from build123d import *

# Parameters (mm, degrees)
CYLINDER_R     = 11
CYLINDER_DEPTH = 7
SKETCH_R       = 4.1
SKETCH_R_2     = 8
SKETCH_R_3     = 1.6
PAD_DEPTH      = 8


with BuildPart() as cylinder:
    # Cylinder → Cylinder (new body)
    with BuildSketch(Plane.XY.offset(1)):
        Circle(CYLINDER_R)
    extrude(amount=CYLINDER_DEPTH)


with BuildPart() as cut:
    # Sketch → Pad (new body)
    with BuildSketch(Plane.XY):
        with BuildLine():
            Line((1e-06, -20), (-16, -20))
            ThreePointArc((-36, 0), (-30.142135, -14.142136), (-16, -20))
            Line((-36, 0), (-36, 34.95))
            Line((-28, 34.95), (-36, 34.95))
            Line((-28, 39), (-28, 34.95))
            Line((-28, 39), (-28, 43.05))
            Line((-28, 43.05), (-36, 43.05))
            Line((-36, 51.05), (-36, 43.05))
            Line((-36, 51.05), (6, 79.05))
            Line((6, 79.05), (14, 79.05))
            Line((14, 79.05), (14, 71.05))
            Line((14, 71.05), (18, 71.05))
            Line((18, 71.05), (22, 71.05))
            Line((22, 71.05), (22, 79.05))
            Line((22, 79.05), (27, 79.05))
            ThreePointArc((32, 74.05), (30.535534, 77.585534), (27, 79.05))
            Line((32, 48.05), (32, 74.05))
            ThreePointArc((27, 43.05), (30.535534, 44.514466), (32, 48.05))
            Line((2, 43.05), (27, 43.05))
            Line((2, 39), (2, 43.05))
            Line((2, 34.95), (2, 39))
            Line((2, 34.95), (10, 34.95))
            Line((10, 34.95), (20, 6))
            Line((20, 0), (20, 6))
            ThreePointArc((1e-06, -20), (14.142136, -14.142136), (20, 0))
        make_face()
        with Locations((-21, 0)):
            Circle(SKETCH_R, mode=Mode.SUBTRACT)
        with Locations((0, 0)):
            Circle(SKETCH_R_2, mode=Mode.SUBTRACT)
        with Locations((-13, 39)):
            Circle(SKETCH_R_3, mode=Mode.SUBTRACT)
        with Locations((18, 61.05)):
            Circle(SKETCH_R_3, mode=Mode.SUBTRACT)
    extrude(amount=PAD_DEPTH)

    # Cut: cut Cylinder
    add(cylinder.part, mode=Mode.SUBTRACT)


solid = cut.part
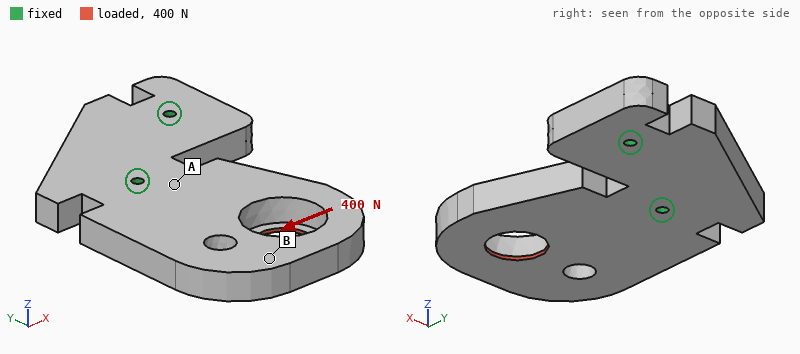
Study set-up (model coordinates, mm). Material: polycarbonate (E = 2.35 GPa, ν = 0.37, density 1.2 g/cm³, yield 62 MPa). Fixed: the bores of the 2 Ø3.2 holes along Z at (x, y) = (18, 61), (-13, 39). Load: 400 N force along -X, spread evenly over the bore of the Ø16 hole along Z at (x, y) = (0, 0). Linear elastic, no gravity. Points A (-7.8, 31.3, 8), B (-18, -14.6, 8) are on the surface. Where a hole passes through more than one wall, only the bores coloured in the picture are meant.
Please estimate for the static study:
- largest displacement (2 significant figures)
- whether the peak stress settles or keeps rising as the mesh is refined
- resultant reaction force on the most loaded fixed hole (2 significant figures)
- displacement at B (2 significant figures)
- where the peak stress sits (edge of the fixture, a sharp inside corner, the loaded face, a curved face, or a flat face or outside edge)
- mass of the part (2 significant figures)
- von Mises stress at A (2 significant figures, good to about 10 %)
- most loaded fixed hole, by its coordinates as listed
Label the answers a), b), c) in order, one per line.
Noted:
a) 0.90 mm
b) keeps rising
c) 750 N
d) 0.67 mm
e) edge of the fixture
f) 42 g
g) 4.1 MPa
h) (-13, 39)
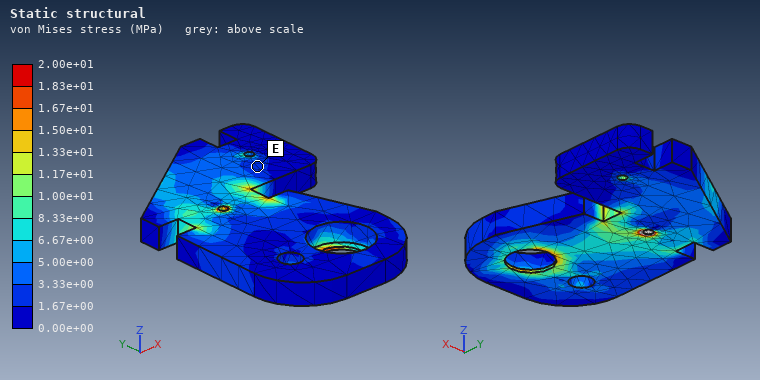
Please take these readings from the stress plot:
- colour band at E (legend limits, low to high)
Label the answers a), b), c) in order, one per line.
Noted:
a) 1.67e+00 to 3.33e+00 MPa
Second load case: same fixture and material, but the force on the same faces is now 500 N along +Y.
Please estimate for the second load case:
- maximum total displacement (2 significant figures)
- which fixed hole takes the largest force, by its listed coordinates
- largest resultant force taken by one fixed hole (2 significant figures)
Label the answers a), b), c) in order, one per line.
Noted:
a) 0.92 mm
b) (-13, 39)
c) 390 N
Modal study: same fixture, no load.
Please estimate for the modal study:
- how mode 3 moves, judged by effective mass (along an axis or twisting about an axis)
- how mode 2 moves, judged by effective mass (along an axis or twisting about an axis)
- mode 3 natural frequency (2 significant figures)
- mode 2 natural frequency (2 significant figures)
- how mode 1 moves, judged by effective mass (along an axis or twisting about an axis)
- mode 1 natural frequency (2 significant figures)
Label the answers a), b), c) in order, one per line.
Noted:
a) along X
b) twisting about Y
c) 1000 Hz
d) 880 Hz
e) along Z
f) 440 Hz
